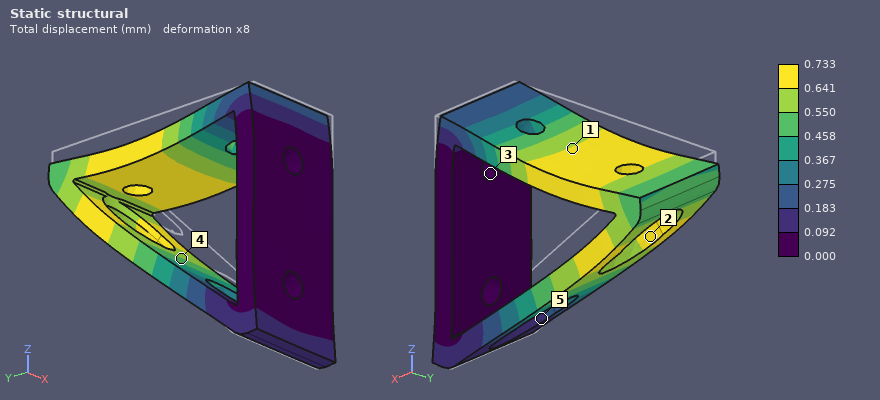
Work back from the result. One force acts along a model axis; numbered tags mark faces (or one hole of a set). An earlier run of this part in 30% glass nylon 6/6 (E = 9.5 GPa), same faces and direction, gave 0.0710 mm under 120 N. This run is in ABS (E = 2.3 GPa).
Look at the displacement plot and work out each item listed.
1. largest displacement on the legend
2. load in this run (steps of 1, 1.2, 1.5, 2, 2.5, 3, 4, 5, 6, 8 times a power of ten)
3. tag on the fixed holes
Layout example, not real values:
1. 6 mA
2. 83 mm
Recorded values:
1. 0.733 mm
2. 300 N
3. 3
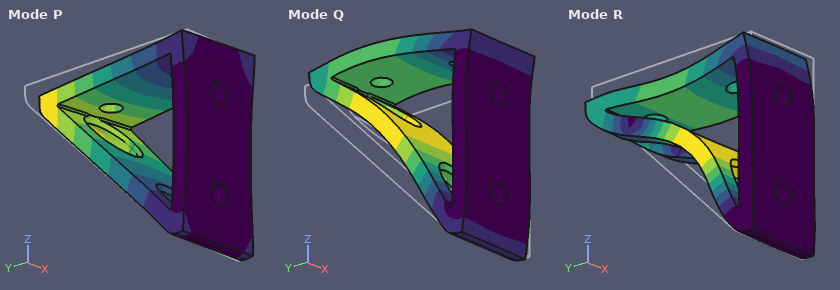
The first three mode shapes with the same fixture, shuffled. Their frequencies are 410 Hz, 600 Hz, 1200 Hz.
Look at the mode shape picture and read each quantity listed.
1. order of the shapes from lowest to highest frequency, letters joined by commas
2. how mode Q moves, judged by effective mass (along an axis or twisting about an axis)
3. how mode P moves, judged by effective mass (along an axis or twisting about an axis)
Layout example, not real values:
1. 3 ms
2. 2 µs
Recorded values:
1. P, Q, R
2. along Z
3. along X
